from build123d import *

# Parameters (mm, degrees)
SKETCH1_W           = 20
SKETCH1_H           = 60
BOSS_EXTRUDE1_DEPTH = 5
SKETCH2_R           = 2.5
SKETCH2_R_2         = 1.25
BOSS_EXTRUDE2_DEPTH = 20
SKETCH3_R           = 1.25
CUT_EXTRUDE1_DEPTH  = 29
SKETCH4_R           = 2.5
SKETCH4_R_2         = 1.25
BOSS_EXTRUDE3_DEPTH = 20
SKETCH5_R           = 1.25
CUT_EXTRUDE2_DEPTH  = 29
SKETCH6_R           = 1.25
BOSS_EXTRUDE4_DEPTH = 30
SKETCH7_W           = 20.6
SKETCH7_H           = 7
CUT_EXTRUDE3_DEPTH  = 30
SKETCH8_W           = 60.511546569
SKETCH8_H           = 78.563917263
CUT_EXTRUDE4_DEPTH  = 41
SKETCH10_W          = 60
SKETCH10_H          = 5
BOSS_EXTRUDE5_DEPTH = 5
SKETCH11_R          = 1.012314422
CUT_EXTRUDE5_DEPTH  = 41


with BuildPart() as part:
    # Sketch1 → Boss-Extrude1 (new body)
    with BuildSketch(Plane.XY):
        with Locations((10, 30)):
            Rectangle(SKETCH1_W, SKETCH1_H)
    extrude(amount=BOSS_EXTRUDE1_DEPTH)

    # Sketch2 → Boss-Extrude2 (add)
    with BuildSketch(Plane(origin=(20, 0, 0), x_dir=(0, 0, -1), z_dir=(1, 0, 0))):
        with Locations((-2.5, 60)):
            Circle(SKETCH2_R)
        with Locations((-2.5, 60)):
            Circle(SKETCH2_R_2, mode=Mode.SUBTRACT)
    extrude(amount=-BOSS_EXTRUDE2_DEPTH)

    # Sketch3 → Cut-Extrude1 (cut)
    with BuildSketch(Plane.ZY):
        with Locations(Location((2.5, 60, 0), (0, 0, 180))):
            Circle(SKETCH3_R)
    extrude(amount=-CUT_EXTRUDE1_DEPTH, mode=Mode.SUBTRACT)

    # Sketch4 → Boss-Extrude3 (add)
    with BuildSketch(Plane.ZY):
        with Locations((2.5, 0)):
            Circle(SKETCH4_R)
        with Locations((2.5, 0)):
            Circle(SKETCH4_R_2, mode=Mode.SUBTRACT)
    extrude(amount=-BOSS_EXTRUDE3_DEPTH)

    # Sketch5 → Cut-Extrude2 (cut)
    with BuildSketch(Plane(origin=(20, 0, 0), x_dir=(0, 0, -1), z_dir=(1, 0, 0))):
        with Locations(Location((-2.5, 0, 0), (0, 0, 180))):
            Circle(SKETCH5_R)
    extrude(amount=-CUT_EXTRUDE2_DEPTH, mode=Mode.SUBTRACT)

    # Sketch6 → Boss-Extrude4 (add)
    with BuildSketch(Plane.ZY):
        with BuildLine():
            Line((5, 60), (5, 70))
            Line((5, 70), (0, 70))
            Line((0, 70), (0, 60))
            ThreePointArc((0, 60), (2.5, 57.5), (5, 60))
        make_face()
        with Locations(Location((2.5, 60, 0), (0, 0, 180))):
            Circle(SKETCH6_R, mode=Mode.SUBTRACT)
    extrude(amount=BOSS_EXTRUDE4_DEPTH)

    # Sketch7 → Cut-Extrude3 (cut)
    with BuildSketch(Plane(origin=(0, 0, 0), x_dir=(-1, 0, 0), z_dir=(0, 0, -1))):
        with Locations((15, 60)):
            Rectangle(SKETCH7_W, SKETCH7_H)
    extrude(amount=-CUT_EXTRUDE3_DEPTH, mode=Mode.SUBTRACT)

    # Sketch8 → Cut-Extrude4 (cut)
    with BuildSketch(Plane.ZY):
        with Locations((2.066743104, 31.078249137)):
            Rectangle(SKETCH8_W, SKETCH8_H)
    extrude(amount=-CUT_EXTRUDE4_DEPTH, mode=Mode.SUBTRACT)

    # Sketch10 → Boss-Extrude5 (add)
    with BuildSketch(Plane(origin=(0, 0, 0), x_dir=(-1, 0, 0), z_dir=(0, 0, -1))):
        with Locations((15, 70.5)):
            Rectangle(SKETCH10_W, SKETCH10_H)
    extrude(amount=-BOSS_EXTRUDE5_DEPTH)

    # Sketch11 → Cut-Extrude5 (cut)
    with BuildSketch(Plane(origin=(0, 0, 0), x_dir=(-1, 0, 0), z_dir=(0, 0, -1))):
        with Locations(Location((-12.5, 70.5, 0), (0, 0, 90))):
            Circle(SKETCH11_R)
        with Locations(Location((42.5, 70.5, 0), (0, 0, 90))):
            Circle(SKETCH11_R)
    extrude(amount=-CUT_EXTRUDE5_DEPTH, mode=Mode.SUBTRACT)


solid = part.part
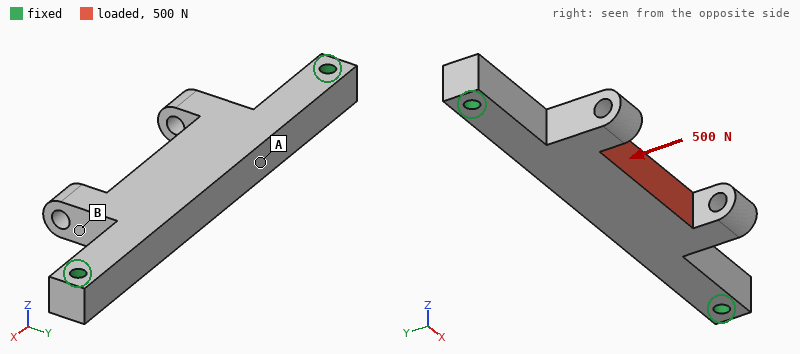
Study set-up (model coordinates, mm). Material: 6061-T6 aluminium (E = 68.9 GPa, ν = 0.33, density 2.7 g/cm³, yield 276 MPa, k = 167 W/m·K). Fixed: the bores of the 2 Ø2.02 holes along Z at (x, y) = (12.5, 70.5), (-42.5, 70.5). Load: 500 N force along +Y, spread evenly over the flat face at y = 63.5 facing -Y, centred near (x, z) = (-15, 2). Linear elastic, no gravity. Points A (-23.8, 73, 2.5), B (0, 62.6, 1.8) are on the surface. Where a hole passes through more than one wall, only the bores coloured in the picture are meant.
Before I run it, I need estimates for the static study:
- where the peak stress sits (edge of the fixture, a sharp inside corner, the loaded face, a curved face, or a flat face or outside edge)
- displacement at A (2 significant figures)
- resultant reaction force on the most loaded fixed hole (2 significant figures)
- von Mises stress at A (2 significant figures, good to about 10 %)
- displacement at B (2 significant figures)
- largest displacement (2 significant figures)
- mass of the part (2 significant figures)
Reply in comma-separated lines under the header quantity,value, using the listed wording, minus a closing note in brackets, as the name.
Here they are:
quantity,value
where the peak stress sits,edge of the fixture
displacement at A,42 µm
resultant reaction force on the most loaded fixed hole,360 N
von Mises stress at A,27 MPa
displacement at B,35 µm
largest displacement,48 µm
mass of the part,6.4 g
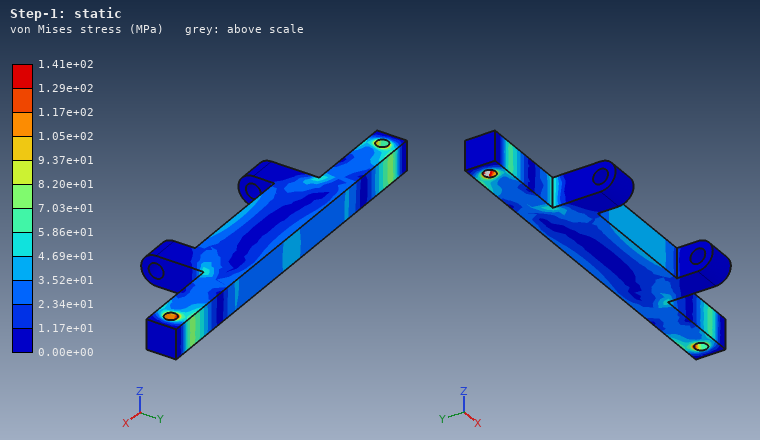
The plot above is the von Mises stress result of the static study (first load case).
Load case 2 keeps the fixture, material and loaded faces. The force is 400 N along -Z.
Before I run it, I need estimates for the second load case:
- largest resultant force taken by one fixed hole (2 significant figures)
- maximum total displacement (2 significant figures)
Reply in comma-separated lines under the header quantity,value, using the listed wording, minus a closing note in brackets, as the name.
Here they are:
quantity,value
largest resultant force taken by one fixed hole,200 N
maximum total displacement,0.16 mm
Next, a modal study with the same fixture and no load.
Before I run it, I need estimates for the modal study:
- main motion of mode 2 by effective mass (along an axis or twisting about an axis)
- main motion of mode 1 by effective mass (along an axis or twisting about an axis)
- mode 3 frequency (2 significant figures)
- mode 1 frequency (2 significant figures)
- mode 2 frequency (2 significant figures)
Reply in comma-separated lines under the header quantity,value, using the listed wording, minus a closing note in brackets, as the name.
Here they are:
quantity,value
main motion of mode 2 by effective mass,along Y
main motion of mode 1 by effective mass,along Z
mode 3 frequency,12 kHz
mode 1 frequency,5900 Hz
mode 2 frequency,8200 Hz
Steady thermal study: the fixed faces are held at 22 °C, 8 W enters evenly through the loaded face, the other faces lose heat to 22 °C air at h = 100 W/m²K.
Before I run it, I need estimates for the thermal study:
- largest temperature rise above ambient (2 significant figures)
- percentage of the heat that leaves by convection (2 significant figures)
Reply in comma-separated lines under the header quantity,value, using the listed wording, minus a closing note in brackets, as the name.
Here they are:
quantity,value
largest temperature rise above ambient,16 K
percentage of the heat that leaves by convection,20 %
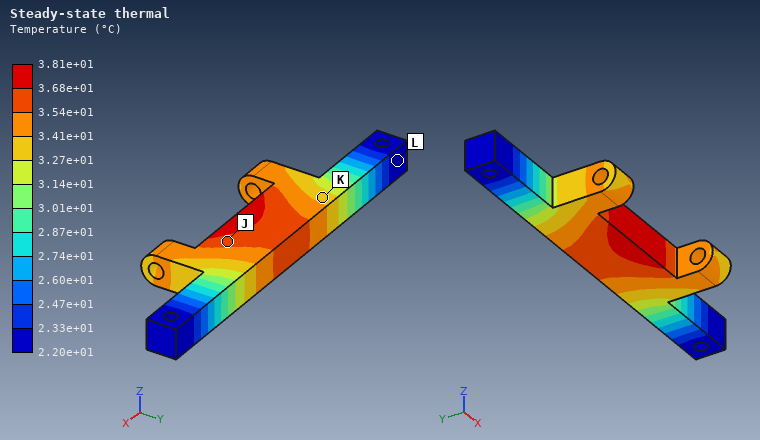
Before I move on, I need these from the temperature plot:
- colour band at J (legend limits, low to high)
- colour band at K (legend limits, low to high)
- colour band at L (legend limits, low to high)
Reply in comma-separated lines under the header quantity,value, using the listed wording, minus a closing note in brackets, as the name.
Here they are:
quantity,value
colour band at J,3.54e+01 to 3.68e+01 °C
colour band at K,3.27e+01 to 3.41e+01 °C
colour band at L,2.20e+01 to 2.33e+01 °C
